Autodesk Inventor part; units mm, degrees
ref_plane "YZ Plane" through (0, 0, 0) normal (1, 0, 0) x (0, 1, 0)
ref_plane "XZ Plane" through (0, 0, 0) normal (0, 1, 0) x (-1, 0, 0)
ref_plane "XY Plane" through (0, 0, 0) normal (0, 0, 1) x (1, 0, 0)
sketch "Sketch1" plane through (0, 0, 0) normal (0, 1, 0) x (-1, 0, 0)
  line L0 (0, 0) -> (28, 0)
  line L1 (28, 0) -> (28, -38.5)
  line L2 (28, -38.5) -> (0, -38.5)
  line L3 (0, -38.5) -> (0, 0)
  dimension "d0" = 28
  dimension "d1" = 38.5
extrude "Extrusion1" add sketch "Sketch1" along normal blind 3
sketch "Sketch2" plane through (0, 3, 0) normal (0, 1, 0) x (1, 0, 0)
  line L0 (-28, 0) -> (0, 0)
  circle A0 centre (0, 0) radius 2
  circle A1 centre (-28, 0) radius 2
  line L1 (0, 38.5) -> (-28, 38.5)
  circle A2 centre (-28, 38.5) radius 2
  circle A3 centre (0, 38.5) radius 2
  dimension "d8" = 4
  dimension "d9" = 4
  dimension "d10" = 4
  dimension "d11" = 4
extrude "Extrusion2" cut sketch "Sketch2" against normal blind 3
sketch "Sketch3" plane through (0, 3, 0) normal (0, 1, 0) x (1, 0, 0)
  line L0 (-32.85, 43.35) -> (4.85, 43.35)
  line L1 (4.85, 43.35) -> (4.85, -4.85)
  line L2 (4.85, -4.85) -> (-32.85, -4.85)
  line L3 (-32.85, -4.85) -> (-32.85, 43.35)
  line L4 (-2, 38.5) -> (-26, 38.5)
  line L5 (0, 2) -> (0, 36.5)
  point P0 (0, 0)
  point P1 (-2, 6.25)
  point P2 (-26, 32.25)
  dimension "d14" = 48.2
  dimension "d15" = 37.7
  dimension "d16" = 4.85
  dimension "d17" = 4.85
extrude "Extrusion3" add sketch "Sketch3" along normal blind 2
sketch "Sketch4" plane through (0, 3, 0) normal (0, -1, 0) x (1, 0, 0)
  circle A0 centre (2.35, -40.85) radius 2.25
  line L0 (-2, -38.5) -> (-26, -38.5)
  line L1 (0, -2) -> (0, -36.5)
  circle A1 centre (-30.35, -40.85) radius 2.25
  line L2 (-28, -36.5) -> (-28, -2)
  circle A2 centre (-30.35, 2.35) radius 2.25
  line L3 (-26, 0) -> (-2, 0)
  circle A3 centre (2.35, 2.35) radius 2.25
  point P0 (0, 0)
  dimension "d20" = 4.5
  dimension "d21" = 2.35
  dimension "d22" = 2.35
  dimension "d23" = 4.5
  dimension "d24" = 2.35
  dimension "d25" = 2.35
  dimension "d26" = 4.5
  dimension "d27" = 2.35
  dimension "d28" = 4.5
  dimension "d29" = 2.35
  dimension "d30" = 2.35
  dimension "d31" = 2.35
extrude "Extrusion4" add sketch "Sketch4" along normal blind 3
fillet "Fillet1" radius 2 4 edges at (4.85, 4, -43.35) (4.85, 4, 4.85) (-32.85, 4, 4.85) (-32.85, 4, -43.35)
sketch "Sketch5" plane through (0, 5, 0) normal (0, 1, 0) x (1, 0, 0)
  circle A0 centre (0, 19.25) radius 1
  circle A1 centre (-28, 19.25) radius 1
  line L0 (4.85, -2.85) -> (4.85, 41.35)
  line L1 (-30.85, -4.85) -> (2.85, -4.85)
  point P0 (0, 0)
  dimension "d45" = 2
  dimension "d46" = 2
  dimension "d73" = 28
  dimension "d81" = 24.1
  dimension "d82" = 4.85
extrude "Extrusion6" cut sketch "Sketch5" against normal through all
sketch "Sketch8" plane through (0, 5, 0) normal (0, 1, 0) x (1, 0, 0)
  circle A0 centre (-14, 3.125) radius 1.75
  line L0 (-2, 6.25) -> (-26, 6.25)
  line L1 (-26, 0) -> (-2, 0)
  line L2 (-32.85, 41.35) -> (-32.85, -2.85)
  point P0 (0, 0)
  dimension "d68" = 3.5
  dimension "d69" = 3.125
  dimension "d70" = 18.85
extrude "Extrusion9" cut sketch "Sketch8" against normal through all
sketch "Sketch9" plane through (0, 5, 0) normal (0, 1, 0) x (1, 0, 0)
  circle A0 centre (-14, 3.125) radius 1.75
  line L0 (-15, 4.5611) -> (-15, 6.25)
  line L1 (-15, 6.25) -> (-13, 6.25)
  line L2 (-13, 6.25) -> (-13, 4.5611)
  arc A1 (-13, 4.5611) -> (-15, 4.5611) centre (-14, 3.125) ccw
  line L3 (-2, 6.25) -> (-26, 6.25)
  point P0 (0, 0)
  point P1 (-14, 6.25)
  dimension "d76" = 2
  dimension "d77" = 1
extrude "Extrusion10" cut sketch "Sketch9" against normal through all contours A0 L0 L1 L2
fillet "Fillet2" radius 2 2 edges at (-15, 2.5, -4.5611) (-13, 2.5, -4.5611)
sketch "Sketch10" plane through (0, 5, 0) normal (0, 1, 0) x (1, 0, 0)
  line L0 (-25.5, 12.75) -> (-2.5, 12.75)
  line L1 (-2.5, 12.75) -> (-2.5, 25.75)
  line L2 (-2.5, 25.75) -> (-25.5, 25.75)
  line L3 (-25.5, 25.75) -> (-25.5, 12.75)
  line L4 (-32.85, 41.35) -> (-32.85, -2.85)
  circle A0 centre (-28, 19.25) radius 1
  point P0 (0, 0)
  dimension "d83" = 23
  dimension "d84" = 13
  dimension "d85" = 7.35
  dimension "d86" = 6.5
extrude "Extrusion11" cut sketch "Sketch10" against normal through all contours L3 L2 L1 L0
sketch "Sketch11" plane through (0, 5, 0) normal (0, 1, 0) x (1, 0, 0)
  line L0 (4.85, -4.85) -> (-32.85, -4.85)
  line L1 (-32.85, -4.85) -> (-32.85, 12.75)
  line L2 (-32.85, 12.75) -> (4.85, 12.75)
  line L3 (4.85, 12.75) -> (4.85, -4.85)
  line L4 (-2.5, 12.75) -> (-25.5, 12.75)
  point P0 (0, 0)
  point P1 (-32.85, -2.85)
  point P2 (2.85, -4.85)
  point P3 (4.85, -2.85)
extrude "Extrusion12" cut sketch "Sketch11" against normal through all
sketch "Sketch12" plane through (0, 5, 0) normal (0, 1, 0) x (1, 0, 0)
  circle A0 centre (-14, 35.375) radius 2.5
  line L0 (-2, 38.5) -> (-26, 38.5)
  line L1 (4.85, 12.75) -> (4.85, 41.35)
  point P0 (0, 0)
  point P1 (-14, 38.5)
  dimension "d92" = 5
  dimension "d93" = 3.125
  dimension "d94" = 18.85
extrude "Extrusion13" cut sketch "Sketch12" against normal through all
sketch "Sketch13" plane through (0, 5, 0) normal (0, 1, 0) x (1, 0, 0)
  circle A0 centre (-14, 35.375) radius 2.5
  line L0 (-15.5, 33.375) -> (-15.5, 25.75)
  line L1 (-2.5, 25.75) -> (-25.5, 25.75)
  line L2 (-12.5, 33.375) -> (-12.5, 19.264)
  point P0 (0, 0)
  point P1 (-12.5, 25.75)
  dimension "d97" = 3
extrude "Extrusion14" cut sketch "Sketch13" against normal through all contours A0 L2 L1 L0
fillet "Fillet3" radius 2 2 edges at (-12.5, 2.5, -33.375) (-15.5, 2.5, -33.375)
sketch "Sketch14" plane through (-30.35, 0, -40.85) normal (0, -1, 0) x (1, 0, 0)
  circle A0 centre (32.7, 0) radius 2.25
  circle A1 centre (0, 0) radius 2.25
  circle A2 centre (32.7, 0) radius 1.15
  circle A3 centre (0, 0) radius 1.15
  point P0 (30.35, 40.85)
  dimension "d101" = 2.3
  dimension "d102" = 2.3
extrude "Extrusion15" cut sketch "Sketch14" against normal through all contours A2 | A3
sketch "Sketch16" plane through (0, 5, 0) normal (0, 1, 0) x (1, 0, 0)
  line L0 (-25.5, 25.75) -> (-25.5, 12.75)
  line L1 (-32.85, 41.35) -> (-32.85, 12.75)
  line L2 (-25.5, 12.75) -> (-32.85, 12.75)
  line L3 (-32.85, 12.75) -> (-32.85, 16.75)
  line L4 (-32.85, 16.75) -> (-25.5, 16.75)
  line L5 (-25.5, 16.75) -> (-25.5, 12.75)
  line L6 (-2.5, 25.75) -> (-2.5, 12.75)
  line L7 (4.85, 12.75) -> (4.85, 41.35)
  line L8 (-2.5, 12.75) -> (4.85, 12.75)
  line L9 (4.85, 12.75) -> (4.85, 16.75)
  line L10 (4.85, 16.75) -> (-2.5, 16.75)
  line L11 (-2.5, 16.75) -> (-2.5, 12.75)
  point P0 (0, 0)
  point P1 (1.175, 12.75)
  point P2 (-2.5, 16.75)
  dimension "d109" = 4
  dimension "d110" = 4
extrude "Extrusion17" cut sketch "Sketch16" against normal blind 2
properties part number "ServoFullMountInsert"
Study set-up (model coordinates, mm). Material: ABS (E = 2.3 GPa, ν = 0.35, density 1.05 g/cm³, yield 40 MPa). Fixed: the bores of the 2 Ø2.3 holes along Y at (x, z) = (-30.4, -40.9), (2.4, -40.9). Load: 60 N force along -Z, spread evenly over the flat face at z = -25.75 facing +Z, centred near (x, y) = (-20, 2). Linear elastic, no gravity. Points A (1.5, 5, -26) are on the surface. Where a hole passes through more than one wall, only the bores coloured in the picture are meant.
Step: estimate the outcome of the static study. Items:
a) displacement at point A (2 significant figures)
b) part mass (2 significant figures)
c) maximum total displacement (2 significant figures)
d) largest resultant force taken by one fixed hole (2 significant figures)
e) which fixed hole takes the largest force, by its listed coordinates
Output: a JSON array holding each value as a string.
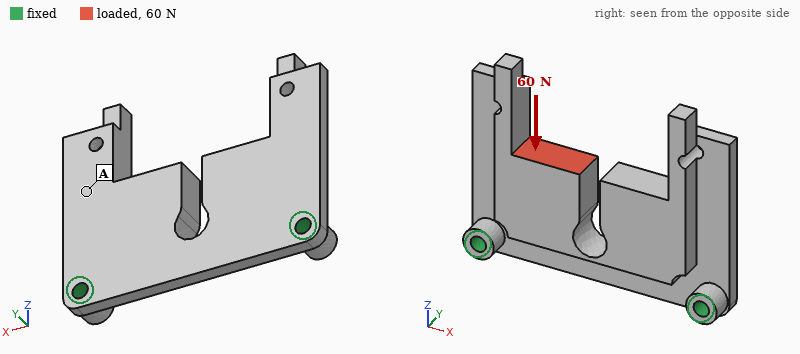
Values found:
["0.12 mm", "2.8 g", "0.50 mm", "45 N", "(-30.4, -40.9)"]
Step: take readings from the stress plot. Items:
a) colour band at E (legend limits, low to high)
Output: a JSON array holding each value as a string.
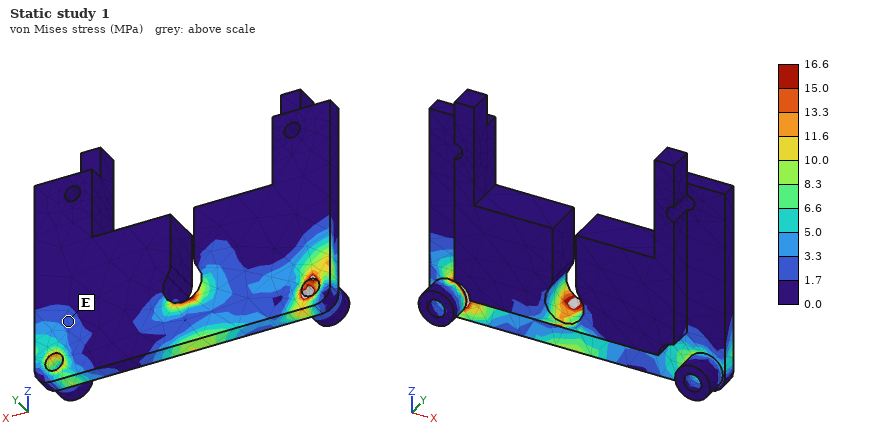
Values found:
["1.7 to 3.3 MPa"]
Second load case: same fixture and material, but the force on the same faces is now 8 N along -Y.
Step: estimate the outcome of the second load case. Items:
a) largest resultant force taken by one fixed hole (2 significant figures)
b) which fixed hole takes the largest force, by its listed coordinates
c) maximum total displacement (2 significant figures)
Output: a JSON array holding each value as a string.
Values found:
["6.7 N", "(-30.4, -40.9)", "0.58 mm"]
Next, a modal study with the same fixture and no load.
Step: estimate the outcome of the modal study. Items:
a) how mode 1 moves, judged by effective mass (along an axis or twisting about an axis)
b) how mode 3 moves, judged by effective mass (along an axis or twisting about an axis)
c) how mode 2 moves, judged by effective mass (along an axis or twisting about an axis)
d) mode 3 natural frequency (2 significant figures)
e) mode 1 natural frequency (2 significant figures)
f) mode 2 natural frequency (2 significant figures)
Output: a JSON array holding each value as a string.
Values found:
["along Y", "along Z", "twisting about Z", "2000 Hz", "820 Hz", "1100 Hz"]
